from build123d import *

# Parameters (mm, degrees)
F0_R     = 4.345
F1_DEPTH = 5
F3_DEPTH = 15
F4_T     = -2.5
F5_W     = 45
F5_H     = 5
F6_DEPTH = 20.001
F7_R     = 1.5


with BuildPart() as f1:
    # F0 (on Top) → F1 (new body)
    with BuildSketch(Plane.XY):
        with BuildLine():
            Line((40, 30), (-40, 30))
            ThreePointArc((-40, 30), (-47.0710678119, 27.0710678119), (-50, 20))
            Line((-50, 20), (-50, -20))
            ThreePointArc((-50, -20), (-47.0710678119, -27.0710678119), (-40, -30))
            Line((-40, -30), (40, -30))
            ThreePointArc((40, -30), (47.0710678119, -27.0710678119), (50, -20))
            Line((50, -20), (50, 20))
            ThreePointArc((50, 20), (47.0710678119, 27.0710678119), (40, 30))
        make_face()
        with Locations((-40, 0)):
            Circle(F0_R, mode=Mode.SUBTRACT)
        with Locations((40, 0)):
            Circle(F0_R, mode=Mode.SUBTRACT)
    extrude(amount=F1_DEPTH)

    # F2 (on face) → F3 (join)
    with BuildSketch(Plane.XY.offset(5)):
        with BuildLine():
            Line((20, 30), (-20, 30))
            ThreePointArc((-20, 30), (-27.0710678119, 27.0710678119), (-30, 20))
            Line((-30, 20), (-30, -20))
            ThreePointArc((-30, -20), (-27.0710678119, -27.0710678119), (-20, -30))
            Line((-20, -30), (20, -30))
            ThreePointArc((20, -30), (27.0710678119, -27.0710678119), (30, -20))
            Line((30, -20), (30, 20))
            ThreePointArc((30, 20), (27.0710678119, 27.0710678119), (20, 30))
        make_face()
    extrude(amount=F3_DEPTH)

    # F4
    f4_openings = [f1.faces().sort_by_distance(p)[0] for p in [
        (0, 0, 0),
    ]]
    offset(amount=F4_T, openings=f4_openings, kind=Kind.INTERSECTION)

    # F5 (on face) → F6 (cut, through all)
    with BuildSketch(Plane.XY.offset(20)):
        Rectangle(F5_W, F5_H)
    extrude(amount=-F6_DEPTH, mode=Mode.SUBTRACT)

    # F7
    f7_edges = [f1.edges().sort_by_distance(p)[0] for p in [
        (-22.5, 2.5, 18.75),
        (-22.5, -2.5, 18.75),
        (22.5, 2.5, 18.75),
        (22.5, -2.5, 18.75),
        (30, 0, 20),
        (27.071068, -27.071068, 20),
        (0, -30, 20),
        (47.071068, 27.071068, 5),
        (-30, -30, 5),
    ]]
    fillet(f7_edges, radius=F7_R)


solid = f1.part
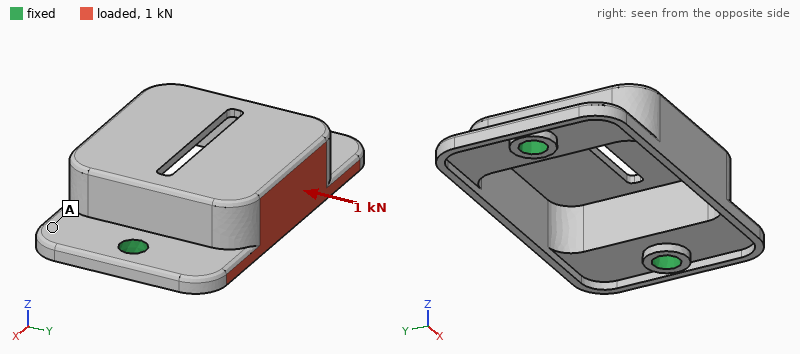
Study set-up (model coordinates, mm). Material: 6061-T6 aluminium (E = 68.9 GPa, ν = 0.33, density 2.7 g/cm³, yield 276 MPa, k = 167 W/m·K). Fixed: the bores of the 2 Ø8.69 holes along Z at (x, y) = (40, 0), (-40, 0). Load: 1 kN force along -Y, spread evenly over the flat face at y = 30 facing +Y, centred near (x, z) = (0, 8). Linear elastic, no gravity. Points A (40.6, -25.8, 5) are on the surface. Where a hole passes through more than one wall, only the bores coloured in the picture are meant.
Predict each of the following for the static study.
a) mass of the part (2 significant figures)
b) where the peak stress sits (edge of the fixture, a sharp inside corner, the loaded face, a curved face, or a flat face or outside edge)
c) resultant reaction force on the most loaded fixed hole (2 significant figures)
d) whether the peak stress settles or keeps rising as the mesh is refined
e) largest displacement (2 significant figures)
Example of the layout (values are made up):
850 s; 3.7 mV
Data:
65 g; a sharp inside corner; 540 N; keeps rising; 0.15 mm
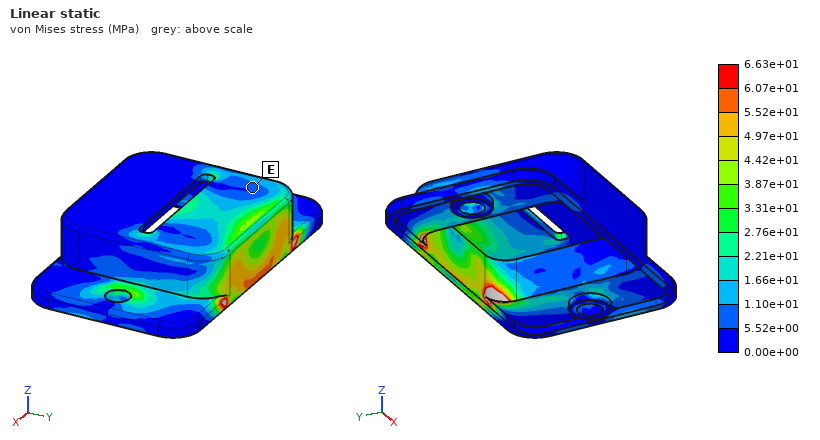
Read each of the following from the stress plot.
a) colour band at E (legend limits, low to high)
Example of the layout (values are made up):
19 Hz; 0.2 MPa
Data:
5.52e+00 to 1.10e+01 MPa
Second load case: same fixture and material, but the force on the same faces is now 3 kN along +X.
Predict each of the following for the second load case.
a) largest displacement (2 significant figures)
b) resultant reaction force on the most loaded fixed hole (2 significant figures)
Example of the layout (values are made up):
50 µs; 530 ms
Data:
0.13 mm; 1.6 kN
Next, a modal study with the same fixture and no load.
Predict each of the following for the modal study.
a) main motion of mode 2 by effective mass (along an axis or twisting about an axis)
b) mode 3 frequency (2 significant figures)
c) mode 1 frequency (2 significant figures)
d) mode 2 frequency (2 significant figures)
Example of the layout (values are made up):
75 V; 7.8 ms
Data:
along Z; 4900 Hz; 1800 Hz; 4400 Hz
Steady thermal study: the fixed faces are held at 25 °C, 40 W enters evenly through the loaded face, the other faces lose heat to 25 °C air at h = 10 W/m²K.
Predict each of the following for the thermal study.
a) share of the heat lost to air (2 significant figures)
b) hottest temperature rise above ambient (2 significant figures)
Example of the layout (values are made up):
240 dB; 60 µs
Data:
7.9 %; 55 K
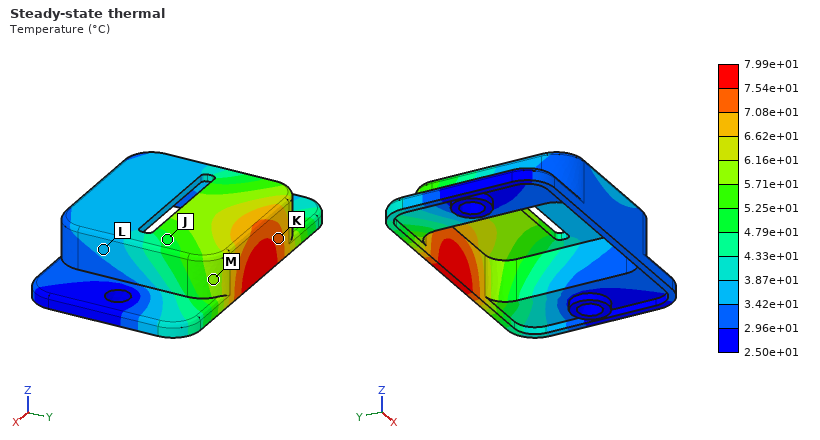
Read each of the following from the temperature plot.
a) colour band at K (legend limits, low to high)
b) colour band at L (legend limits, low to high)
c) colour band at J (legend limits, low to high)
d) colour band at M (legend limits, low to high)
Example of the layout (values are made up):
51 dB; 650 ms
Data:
7.08e+01 to 7.54e+01 °C; 3.42e+01 to 3.87e+01 °C; 4.79e+01 to 5.25e+01 °C; 5.71e+01 to 6.16e+01 °C
